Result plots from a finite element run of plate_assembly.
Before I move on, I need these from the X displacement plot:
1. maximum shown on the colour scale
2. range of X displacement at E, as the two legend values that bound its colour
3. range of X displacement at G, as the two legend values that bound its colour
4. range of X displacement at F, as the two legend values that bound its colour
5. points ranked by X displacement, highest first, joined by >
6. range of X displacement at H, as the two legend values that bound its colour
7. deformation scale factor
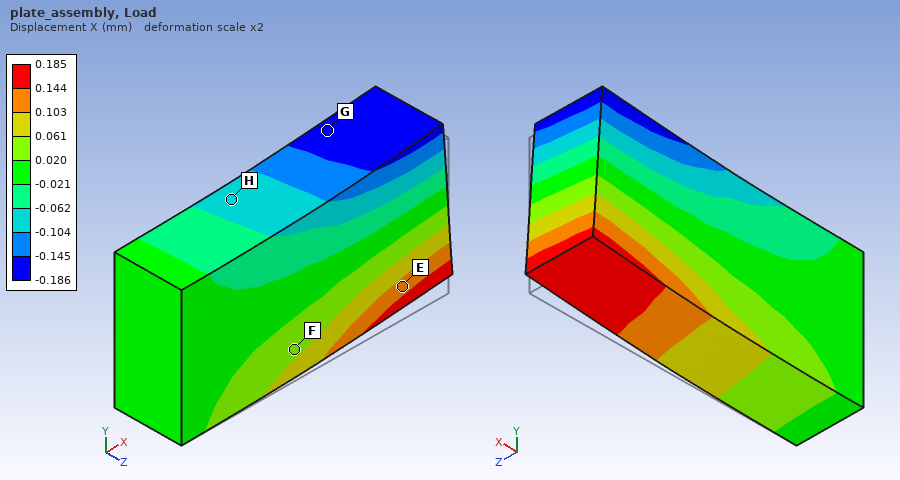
0.185 mm
0.103 to 0.144 mm
-0.186 to -0.145 mm
0.020 to 0.061 mm
E > F > H > G
-0.104 to -0.062 mm
2
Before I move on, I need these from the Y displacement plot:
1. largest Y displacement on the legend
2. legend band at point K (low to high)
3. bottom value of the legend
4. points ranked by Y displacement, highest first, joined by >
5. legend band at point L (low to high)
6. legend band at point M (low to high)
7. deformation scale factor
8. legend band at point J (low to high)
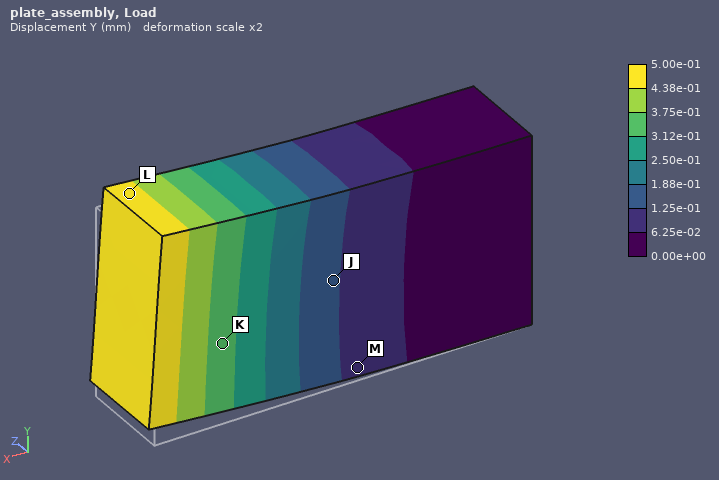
5.00e-01 mm
3.12e-01 to 3.75e-01 mm
0.00e+00 mm
L > K > J > M
4.38e-01 to 5.00e-01 mm
6.25e-02 to 1.25e-01 mm
2
1.25e-01 to 1.88e-01 mm
